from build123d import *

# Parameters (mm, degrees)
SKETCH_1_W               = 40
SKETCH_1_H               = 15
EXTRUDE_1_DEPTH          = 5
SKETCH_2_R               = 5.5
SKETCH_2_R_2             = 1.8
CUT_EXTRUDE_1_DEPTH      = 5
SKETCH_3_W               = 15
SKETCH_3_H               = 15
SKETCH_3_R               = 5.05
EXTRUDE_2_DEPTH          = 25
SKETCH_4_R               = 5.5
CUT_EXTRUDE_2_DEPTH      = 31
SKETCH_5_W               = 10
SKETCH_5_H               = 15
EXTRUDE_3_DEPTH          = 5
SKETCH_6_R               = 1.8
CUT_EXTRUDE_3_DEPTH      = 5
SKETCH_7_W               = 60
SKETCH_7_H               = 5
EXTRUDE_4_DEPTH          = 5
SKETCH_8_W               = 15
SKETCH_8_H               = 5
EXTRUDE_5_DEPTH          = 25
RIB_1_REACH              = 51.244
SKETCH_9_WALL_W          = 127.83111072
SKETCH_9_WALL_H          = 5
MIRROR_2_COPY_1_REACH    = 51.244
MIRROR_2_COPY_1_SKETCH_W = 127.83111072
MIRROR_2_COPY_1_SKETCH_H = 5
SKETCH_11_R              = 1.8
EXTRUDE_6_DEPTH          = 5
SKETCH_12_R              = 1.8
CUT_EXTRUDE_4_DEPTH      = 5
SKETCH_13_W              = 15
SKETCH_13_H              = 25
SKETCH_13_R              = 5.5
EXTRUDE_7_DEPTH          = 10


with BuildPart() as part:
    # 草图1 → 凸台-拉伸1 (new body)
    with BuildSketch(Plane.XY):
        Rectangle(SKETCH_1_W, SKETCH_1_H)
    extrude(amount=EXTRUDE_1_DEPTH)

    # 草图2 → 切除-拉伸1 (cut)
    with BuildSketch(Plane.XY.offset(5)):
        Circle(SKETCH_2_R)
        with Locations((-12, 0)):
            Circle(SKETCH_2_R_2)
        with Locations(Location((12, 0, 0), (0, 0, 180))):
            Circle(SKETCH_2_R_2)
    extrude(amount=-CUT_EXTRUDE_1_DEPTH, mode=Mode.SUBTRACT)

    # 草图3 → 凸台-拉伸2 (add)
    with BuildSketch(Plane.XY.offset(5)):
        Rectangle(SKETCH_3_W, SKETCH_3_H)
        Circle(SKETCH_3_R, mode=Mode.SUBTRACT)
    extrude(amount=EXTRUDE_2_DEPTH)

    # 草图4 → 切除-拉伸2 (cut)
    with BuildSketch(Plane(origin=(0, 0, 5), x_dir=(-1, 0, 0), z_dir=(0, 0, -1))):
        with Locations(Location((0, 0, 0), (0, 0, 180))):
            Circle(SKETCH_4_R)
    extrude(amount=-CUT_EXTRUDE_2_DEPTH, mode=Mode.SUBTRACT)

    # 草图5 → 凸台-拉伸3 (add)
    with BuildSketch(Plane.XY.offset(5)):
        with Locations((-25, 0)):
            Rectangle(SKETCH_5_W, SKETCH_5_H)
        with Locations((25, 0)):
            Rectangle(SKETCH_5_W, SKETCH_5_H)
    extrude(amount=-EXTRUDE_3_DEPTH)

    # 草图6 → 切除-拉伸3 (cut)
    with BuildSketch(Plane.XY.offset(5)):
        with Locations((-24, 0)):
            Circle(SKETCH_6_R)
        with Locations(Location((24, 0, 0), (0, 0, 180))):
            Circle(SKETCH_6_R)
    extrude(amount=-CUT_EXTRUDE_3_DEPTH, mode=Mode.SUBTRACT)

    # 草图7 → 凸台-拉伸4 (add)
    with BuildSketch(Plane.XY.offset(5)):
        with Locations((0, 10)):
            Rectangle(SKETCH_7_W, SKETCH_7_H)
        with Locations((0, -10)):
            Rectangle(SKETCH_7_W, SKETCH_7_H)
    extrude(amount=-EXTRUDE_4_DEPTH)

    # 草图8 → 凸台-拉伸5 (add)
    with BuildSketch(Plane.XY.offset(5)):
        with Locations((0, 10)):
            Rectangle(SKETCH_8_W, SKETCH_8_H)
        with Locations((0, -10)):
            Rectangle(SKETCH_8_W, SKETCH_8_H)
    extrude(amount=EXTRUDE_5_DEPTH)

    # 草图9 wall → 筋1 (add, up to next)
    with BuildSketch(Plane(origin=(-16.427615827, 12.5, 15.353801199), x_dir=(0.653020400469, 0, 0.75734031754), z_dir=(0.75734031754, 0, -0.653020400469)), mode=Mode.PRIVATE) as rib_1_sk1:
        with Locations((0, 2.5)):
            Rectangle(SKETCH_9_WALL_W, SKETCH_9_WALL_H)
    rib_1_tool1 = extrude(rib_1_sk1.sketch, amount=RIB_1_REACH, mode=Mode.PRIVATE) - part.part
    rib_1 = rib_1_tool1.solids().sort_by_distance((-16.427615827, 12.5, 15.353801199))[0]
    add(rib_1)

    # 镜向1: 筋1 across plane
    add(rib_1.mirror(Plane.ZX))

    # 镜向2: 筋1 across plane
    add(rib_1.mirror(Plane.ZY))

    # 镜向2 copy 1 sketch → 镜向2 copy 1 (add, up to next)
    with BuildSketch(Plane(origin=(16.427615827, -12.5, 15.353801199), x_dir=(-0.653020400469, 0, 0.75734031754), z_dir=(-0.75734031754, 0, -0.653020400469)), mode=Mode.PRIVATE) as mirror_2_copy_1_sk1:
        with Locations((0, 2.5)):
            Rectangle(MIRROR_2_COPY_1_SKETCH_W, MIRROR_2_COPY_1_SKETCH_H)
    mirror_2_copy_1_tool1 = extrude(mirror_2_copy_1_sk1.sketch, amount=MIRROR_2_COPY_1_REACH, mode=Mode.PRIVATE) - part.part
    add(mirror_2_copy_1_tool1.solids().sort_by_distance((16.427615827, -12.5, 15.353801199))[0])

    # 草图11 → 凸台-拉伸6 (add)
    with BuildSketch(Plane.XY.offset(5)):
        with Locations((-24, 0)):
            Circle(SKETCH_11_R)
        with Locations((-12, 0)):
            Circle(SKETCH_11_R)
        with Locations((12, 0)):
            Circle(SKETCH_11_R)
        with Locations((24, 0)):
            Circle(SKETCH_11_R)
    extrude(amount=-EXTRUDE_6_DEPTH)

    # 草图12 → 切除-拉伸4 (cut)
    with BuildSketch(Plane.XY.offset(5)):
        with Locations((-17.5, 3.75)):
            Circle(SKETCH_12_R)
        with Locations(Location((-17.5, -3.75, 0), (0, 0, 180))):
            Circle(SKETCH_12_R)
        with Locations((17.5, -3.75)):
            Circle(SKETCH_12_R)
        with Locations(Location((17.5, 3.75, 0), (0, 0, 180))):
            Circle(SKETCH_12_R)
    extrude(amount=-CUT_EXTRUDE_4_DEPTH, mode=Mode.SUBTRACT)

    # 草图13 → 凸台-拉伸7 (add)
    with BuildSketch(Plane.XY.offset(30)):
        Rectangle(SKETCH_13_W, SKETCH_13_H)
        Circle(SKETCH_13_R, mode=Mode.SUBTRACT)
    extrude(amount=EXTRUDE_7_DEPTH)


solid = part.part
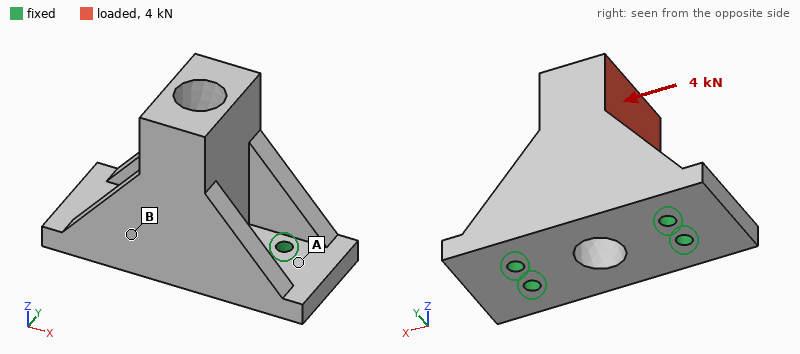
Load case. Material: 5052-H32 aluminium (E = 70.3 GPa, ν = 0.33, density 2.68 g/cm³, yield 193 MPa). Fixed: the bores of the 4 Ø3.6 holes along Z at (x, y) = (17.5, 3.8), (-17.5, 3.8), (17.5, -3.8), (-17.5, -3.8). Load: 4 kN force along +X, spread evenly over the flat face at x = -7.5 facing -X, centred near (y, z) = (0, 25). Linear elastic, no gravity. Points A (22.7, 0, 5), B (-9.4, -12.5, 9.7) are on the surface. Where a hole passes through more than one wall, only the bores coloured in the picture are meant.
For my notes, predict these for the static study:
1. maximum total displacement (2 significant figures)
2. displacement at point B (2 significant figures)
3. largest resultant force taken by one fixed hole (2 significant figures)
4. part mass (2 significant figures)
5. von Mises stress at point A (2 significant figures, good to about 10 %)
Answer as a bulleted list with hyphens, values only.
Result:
- 49 µm
- 8.2 µm
- 1.6 kN
- 54 g
- 22 MPa
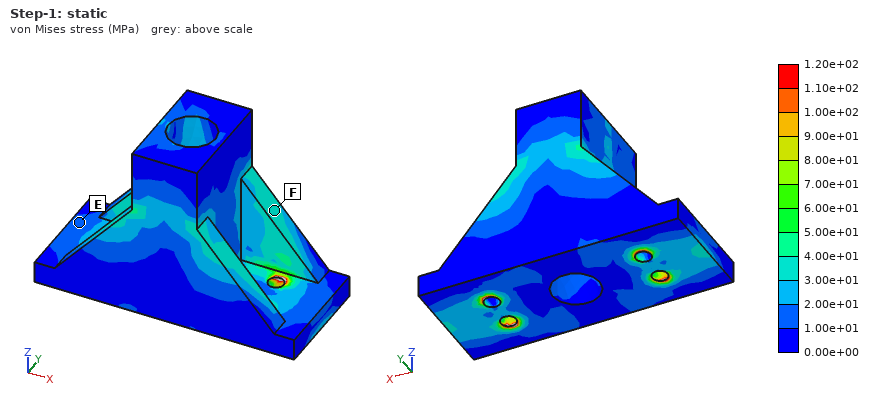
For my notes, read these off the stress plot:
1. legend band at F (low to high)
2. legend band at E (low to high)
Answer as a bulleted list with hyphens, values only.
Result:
- 3.00e+01 to 4.00e+01 MPa
- 1.00e+01 to 2.00e+01 MPa
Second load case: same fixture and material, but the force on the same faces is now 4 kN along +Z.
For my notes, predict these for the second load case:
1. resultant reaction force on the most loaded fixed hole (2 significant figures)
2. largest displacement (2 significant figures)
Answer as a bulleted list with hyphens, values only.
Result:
- 1.5 kN
- 30 µm
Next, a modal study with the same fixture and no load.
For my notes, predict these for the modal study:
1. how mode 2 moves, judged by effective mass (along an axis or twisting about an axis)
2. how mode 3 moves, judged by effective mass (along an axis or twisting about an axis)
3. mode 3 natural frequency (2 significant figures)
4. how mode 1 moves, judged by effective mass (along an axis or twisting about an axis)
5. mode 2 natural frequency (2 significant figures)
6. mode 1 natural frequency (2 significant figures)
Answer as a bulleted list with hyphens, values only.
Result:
- along X
- along Z
- 16 kHz
- along Y
- 12 kHz
- 5400 Hz
